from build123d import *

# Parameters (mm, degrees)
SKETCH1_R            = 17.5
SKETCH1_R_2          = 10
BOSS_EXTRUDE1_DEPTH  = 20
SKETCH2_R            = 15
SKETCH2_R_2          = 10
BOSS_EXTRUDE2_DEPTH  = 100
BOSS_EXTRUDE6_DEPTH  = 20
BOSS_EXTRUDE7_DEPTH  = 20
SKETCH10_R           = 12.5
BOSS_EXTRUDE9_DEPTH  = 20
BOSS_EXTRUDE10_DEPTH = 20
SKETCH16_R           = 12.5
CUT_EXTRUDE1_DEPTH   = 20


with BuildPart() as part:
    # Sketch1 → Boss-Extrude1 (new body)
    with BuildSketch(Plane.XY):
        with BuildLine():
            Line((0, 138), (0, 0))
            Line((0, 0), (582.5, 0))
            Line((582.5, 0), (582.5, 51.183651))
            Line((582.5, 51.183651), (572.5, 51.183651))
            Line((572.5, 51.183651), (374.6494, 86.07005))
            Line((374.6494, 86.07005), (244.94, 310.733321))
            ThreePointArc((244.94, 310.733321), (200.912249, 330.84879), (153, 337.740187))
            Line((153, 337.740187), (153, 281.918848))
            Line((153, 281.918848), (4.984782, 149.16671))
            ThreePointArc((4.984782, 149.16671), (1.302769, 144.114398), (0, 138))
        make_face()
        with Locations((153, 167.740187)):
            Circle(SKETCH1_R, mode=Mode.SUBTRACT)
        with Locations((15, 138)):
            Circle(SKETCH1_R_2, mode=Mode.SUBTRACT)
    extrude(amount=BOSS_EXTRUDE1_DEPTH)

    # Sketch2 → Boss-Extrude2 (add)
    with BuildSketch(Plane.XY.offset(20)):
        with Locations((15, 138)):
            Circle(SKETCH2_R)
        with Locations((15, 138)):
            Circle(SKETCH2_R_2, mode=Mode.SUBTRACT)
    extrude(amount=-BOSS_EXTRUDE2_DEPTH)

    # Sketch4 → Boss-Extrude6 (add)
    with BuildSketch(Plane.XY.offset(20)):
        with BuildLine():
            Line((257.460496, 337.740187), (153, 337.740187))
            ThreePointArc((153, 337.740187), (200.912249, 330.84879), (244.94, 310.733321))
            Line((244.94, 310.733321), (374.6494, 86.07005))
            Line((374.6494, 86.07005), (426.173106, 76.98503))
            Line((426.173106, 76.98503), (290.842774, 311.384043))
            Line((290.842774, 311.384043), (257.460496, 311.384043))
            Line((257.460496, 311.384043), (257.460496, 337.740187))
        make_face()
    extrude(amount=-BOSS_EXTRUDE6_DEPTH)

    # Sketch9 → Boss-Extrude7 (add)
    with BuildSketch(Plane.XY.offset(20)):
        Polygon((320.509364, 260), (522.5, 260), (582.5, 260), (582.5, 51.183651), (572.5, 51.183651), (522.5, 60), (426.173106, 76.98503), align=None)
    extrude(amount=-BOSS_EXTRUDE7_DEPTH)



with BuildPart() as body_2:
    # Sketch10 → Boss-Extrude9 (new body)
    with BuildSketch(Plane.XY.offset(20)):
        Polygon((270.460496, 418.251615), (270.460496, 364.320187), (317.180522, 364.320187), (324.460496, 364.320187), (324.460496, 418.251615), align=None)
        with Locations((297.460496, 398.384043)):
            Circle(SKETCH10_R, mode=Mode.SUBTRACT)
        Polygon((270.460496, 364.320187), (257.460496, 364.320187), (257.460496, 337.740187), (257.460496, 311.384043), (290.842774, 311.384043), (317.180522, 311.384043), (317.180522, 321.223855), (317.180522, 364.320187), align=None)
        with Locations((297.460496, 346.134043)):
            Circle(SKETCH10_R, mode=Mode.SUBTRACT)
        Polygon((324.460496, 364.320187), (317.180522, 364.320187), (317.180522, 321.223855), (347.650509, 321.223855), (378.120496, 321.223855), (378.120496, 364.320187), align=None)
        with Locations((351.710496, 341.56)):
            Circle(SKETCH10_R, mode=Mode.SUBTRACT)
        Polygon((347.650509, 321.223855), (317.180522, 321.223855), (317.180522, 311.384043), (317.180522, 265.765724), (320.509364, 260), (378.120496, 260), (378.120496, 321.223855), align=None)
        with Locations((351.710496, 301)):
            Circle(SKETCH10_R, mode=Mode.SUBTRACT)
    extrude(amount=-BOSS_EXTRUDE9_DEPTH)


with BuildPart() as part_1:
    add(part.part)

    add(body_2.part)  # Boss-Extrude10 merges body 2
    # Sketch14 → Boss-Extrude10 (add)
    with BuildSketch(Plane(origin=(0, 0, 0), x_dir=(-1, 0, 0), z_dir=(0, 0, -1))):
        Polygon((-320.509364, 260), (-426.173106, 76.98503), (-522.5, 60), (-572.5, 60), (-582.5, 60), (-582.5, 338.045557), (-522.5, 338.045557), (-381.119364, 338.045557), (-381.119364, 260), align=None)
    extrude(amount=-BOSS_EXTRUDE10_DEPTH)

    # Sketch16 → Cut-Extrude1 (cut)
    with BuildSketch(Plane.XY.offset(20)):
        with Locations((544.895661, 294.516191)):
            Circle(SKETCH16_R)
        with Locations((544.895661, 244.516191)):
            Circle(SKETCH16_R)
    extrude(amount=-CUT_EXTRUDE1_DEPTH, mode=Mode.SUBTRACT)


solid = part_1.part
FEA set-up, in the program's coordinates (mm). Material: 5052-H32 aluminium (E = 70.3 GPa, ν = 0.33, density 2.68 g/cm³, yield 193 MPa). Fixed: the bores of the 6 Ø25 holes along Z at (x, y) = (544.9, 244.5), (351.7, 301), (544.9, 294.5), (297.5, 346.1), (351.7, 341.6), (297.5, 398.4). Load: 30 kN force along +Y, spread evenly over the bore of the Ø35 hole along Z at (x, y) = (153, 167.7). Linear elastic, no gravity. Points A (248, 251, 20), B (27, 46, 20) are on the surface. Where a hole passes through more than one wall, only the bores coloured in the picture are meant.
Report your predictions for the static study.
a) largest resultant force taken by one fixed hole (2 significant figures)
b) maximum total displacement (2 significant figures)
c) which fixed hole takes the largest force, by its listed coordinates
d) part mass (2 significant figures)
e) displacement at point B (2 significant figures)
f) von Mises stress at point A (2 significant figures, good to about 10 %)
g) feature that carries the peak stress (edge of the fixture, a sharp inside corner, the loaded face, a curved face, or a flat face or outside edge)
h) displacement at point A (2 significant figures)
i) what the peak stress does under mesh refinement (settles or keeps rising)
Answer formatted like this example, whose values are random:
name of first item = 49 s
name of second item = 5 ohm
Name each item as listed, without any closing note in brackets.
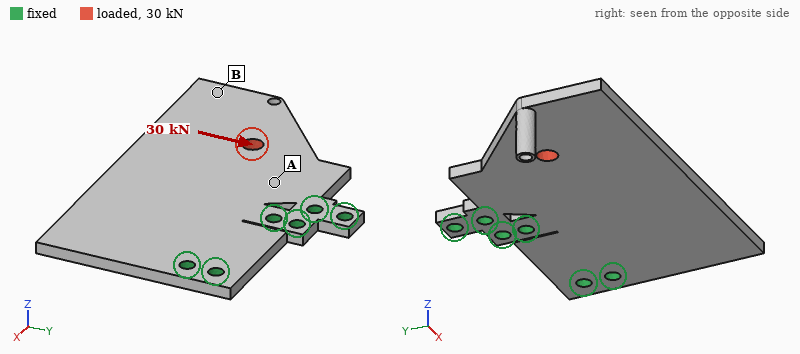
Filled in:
largest resultant force taken by one fixed hole = 26 kN
maximum total displacement = 0.15 mm
which fixed hole takes the largest force, by its listed coordinates = (297.5, 346.1)
part mass = 9.7 kg
displacement at point B = 0.14 mm
von Mises stress at point A = 13 MPa
feature that carries the peak stress = edge of the fixture
displacement at point A = 0.041 mm
what the peak stress does under mesh refinement = keeps rising
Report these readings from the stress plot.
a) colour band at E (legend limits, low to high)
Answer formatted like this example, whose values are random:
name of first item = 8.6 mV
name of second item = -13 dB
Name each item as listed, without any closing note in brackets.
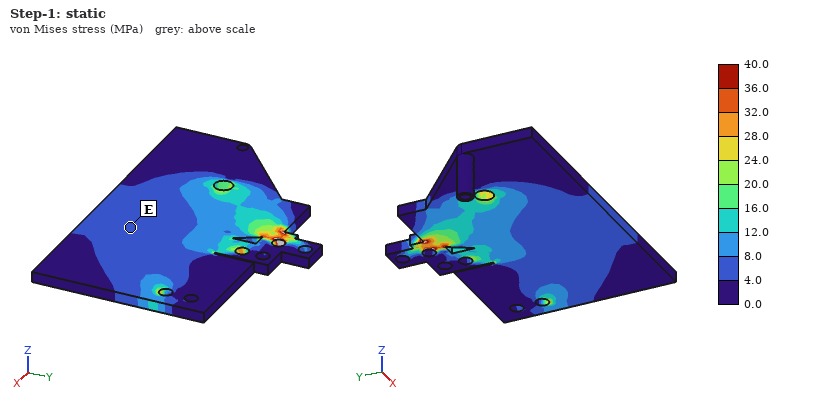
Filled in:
colour band at E = 4.0 to 8.0 MPa
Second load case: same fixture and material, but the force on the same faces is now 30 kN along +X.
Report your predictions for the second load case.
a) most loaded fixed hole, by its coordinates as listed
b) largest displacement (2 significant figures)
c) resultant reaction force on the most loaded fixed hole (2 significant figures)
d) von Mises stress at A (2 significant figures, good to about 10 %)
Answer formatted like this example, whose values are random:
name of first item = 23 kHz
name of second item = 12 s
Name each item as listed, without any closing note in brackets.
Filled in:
most loaded fixed hole, by its coordinates as listed = (544.9, 244.5)
largest displacement = 74 µm
resultant reaction force on the most loaded fixed hole = 18 kN
von Mises stress at A = 6.6 MPa
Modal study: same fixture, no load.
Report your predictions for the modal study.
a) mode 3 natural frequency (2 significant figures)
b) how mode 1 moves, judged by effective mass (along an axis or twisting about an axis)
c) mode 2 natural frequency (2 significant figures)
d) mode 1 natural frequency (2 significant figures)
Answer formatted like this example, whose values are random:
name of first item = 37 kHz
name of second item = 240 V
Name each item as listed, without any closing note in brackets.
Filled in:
mode 3 natural frequency = 500 Hz
how mode 1 moves, judged by effective mass = along Z
mode 2 natural frequency = 250 Hz
mode 1 natural frequency = 100 Hz
